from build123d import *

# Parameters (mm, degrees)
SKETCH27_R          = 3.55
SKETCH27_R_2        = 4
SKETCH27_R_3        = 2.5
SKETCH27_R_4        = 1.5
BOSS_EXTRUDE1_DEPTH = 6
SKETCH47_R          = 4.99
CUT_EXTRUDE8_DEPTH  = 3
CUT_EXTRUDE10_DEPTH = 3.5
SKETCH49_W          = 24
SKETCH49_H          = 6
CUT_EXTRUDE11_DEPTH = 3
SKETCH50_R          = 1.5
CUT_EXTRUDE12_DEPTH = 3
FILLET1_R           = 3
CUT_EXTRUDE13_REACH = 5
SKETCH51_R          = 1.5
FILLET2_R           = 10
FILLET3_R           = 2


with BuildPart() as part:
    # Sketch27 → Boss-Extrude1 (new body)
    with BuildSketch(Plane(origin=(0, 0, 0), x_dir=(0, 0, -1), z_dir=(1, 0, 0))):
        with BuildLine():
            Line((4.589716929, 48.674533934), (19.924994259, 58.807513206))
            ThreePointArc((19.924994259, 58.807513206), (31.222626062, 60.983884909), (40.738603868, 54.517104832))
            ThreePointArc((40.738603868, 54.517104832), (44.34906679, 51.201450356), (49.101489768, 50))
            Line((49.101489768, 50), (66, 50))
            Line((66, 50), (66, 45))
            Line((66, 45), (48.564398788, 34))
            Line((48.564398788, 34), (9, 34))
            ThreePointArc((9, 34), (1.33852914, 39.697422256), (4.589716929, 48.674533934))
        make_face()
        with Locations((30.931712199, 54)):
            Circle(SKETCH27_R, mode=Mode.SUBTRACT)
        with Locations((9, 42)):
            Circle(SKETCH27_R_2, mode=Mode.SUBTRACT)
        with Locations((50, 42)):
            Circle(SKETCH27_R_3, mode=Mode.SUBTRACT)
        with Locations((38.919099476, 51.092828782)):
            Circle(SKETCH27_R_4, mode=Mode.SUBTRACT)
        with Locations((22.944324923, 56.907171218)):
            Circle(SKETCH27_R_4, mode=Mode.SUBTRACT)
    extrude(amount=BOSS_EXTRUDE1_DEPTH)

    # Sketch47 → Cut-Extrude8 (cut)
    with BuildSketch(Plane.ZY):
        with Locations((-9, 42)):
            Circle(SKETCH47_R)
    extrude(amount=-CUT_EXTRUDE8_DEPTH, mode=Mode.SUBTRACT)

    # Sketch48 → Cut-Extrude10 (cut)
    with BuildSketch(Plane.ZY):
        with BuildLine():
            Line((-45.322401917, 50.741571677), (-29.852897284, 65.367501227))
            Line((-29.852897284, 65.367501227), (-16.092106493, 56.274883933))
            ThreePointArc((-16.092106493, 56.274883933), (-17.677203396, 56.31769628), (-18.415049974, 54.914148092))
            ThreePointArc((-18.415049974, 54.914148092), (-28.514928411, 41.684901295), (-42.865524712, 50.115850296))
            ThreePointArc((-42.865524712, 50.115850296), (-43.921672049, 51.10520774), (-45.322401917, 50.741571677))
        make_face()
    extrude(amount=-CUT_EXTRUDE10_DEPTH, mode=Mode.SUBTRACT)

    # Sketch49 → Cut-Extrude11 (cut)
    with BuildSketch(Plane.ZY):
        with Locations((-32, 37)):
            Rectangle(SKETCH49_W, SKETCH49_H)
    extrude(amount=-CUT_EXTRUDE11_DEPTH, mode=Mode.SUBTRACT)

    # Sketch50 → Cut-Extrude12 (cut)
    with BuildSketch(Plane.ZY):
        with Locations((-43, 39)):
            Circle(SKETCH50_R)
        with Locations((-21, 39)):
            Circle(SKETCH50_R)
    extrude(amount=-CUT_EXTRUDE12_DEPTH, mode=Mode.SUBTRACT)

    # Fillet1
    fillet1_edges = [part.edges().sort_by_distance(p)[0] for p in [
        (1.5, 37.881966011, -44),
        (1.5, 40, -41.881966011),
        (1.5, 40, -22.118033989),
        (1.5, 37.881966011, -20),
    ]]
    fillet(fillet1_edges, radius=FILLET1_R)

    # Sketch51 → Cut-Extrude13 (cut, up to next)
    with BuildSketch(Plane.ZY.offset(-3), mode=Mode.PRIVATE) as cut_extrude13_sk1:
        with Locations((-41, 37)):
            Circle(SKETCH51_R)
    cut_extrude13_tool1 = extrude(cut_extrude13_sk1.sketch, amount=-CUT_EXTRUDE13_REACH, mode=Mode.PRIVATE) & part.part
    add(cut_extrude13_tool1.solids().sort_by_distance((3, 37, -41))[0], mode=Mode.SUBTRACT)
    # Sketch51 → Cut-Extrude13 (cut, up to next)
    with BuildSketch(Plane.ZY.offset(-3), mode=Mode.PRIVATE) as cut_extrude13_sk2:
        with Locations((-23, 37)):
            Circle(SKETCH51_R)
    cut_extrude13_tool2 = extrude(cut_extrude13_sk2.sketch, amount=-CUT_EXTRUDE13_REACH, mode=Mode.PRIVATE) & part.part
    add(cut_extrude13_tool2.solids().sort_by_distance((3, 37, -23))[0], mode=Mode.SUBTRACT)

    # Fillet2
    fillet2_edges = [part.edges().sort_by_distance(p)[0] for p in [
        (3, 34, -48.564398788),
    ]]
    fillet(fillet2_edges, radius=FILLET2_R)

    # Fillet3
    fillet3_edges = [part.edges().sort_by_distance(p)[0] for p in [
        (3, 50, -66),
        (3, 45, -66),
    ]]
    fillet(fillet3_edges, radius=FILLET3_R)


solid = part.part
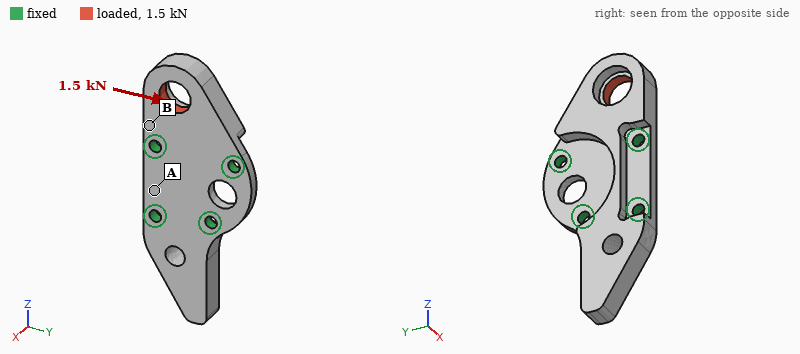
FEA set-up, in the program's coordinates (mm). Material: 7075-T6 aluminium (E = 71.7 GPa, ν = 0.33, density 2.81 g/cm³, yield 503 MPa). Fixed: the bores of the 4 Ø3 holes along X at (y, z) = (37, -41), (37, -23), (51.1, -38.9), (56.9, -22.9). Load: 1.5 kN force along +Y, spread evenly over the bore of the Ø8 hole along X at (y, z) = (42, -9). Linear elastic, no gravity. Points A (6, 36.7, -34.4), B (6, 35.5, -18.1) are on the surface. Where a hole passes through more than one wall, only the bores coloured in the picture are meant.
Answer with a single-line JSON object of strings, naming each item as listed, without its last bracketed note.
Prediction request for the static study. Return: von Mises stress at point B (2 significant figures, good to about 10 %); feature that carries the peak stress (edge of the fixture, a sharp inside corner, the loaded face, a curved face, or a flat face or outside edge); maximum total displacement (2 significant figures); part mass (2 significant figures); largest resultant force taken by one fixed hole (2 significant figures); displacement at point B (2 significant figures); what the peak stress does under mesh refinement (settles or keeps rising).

{"von Mises stress at point B": "50 MPa", "feature that carries the peak stress": "edge of the fixture", "maximum total displacement": "38 µm", "part mass": "13 g", "largest resultant force taken by one fixed hole": "1.3 kN", "displacement at point B": "7.4 µm", "what the peak stress does under mesh refinement": "keeps rising"}
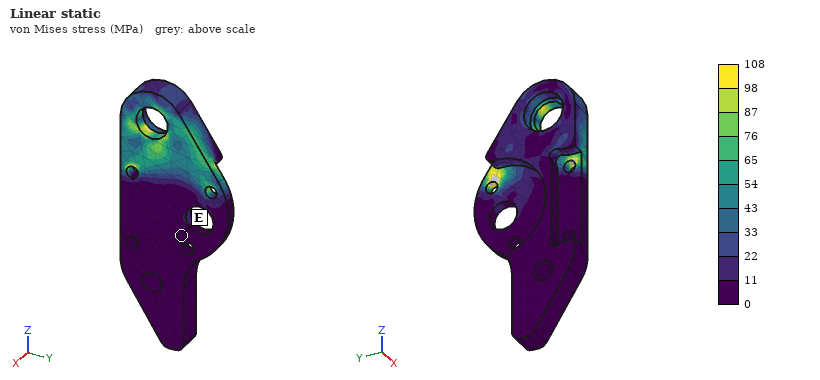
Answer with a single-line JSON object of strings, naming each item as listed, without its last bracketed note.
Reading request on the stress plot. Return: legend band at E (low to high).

{"legend band at E": "0 to 11 MPa"}
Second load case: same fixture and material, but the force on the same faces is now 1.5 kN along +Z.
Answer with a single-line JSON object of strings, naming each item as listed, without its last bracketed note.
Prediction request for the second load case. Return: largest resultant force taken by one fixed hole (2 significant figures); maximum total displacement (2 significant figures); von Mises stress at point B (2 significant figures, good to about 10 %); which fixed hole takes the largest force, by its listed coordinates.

{"largest resultant force taken by one fixed hole": "990 N", "maximum total displacement": "21 µm", "von Mises stress at point B": "50 MPa", "which fixed hole takes the largest force, by its listed coordinates": "(37, -23)"}
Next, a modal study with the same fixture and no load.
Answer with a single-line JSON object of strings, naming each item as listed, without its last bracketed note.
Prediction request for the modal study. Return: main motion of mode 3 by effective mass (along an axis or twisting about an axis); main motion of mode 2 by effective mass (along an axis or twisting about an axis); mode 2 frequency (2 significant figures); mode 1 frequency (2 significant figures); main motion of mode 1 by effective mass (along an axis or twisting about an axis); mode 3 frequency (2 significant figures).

{"main motion of mode 3 by effective mass": "along Y", "main motion of mode 2 by effective mass": "along X", "mode 2 frequency": "7200 Hz", "mode 1 frequency": "6000 Hz", "main motion of mode 1 by effective mass": "along X", "mode 3 frequency": "18 kHz"}
